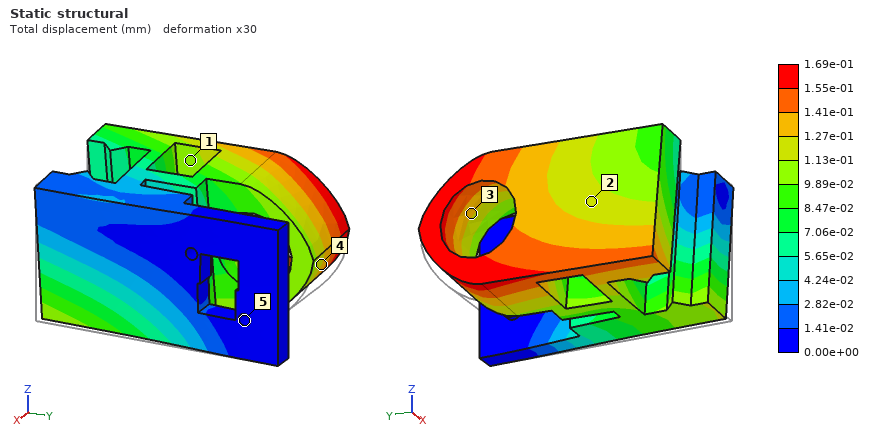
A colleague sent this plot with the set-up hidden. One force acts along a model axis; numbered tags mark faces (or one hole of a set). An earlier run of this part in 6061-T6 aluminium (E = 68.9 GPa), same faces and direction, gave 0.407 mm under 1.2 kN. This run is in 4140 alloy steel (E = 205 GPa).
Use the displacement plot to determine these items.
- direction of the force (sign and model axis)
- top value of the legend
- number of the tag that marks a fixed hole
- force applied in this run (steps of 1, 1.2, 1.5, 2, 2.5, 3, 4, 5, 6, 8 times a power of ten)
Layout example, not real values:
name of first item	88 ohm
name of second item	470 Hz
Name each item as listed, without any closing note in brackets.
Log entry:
direction of the force	+Z
top value of the legend	1.69e-01 mm
number of the tag that marks a fixed hole	5
force applied in this run	1.5 kN
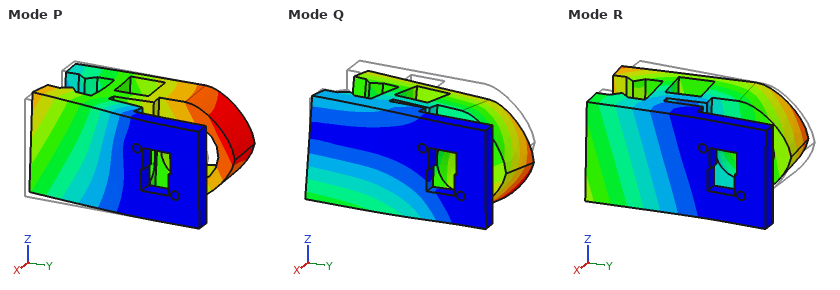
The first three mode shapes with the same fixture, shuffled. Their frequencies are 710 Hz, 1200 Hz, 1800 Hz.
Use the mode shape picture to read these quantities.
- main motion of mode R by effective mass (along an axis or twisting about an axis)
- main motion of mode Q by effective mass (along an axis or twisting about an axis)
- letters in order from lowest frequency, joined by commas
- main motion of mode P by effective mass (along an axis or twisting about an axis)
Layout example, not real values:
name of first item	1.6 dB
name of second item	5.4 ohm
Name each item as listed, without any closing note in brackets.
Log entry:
main motion of mode R by effective mass	along Y
main motion of mode Q by effective mass	along Z
letters in order from lowest frequency, joined by commas	R, Q, P
main motion of mode P by effective mass	along X
